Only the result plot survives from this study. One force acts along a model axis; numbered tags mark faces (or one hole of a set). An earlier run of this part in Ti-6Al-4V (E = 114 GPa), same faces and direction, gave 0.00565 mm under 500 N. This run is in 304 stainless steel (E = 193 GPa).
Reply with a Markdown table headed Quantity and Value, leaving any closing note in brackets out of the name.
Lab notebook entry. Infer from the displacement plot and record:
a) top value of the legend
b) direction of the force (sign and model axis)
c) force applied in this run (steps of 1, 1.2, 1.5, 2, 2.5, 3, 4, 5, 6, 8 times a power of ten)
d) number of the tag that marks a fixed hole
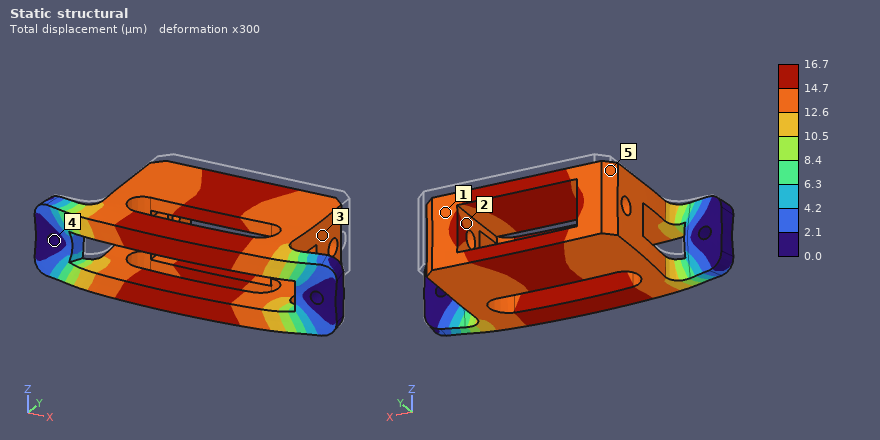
| Quantity | Value |
|---|---|
| top value of the legend | 16.7 µm |
| direction of the force | -Y |
| force applied in this run | 2.5 kN |
| number of the tag that marks a fixed hole | 4 |
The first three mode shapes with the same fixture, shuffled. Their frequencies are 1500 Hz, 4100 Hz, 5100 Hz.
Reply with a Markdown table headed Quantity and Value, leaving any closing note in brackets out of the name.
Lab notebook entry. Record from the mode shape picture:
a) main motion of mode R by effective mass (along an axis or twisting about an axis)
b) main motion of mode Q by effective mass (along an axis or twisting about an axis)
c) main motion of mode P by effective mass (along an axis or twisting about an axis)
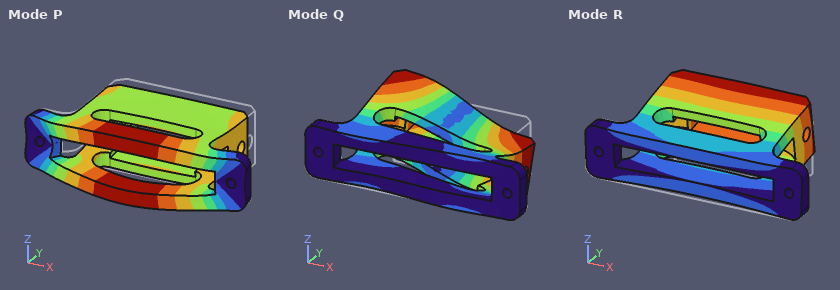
| Quantity | Value |
|---|---|
| main motion of mode R by effective mass | along Z |
| main motion of mode Q by effective mass | twisting about Y |
| main motion of mode P by effective mass | along Y |
